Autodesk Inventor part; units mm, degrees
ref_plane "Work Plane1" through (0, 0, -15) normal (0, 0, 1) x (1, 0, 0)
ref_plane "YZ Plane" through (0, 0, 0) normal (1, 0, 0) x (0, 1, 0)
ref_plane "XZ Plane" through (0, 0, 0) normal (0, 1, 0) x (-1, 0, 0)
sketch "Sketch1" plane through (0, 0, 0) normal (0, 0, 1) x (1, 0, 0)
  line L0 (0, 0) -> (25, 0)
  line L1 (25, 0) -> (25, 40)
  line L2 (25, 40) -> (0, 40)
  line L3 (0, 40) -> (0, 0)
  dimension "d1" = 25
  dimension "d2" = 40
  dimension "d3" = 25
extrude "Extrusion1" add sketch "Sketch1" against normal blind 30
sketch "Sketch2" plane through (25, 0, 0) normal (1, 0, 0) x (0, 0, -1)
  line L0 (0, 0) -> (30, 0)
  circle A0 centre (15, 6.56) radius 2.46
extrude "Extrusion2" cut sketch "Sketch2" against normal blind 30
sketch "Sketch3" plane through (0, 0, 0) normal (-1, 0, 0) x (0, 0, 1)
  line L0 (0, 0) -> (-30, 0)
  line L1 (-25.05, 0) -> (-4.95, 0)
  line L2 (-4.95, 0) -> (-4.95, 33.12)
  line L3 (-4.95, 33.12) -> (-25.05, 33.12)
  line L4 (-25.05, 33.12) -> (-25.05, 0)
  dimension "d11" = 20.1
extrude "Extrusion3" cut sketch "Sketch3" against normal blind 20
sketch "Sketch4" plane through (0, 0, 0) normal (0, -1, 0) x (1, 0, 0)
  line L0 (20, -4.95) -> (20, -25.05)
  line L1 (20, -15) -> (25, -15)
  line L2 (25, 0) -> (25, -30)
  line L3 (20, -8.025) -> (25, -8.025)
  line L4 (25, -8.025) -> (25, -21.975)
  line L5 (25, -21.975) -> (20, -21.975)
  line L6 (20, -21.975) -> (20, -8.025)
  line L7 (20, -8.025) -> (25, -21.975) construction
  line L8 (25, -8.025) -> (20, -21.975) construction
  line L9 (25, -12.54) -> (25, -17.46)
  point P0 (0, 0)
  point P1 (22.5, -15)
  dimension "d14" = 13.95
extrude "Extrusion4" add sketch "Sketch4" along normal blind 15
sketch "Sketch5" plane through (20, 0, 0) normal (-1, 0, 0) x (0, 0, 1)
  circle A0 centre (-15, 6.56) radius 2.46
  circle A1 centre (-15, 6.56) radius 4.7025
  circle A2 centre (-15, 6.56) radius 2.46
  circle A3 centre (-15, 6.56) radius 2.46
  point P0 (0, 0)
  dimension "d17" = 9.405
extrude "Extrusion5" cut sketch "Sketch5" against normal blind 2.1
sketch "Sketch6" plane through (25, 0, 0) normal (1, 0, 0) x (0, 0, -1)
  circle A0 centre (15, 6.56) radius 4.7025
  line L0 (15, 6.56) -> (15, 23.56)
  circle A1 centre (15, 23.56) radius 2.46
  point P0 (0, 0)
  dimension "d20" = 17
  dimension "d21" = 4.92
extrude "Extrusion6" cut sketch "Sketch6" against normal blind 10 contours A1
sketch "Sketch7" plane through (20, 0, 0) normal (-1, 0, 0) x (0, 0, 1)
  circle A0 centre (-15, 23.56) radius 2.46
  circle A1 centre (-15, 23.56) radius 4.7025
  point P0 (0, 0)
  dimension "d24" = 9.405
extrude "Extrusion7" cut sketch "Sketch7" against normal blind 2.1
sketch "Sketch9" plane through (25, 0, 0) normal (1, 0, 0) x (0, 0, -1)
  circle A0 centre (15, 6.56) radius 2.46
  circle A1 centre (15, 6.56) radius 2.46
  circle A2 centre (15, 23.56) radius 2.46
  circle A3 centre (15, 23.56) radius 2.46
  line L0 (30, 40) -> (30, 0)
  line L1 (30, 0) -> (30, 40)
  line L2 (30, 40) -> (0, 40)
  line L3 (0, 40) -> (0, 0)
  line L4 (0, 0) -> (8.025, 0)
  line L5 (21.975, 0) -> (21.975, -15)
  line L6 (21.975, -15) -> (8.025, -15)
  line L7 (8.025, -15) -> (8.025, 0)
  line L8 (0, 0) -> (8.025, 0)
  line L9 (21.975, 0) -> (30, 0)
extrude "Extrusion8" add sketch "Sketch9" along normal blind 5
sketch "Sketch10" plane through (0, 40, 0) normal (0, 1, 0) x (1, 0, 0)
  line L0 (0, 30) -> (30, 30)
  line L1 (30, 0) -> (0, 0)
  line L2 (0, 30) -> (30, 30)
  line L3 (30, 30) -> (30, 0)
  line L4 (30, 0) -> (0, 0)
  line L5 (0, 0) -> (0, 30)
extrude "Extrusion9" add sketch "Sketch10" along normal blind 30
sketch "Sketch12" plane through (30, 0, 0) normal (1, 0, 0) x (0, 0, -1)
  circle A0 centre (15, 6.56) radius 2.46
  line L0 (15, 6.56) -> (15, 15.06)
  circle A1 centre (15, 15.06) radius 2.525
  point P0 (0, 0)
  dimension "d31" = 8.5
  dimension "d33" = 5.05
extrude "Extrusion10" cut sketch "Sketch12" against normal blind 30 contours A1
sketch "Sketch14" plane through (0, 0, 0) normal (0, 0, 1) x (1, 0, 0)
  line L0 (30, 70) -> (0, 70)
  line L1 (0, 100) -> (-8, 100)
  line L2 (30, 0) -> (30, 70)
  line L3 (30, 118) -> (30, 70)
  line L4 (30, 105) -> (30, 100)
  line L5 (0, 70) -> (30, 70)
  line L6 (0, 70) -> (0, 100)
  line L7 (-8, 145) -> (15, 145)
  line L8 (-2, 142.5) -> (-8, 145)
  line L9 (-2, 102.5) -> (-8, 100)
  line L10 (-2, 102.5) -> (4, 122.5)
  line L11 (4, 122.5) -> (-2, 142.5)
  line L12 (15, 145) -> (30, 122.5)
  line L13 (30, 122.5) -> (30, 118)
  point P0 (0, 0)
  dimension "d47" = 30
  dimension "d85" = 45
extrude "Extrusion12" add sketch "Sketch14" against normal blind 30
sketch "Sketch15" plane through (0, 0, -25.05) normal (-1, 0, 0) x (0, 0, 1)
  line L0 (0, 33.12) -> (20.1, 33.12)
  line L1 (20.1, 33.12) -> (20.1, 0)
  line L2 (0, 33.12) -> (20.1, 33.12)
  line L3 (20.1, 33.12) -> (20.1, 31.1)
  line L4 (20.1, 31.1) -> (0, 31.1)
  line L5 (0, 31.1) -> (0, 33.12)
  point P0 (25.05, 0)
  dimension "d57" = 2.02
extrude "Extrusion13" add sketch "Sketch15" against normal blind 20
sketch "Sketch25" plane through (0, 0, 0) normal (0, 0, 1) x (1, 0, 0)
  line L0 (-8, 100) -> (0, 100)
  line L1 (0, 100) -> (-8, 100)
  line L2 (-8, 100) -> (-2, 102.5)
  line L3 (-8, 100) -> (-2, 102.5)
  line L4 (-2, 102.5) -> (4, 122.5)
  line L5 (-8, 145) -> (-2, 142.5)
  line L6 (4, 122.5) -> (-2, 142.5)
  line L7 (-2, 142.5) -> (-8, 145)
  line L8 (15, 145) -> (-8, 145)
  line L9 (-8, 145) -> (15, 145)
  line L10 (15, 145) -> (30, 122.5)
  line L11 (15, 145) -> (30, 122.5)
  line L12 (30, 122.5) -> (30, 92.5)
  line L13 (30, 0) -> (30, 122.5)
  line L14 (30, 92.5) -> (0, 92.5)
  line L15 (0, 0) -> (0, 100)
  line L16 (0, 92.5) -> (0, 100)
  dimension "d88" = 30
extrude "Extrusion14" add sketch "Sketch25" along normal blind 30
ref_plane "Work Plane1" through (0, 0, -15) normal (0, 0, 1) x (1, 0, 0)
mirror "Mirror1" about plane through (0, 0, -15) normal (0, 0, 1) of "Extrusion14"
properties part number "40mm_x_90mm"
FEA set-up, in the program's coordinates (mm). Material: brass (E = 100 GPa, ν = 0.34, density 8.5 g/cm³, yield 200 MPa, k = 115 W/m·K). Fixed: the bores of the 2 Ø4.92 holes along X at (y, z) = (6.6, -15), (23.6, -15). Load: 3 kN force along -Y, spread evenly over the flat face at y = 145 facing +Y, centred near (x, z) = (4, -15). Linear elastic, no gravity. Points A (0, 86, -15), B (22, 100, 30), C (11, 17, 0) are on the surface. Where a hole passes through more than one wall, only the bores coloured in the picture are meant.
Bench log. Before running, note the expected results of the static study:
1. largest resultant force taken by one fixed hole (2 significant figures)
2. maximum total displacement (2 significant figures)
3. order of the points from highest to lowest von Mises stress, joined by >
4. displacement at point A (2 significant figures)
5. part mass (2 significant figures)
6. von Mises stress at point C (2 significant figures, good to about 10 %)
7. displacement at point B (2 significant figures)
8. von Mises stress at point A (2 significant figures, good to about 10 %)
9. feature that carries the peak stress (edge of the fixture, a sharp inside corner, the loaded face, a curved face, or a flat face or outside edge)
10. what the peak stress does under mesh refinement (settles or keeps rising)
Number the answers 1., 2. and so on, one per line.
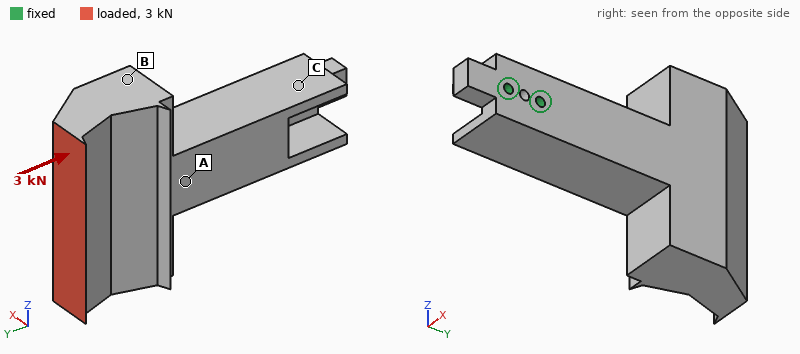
1. 3.1 kN
2. 0.16 mm
3. C > A > B
4. 0.077 mm
5. 1.7 kg
6. 19 MPa
7. 0.087 mm
8. 9.5 MPa
9. edge of the fixture
10. keeps rising
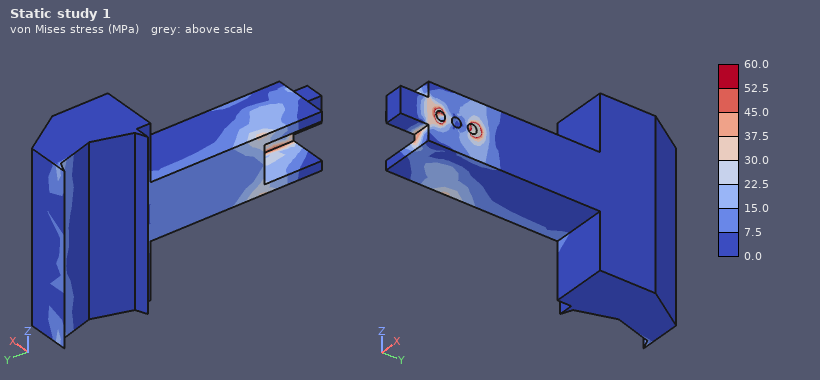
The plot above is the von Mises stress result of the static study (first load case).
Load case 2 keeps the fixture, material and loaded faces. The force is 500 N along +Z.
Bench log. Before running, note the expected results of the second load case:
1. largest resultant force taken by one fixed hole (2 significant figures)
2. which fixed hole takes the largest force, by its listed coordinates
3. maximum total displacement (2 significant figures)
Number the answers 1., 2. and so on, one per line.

1. 3.1 kN
2. (23.6, -15)
3. 0.13 mm
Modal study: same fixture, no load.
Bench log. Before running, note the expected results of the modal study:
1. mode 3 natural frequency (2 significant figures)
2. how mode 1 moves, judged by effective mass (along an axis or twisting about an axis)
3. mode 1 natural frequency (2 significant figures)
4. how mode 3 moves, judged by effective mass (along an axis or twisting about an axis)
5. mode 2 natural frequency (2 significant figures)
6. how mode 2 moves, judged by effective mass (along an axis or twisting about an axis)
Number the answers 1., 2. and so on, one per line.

1. 780 Hz
2. along X
3. 350 Hz
4. twisting about Y
5. 400 Hz
6. along Z
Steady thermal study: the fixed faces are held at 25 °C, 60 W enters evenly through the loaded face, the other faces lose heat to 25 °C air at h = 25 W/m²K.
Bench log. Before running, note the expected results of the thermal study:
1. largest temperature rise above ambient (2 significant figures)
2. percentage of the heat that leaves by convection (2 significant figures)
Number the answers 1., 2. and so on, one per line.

1. 56 K
2. 38 %
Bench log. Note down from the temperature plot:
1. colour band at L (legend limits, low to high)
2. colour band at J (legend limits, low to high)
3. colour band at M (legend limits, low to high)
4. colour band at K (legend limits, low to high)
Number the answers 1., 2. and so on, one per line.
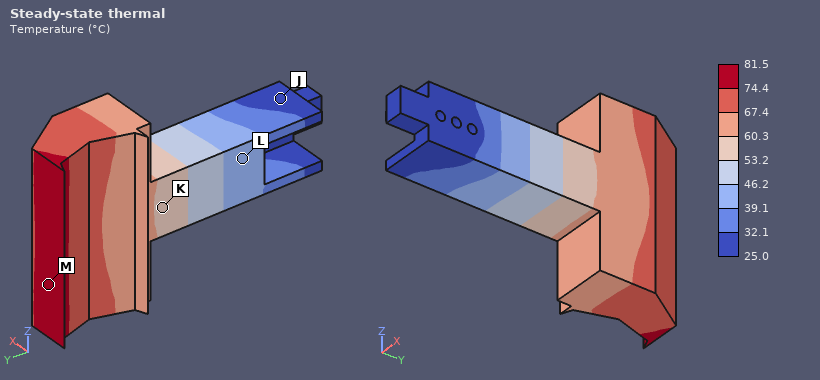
1. 39.1 to 46.2 °C
2. 25.0 to 32.1 °C
3. 74.4 to 81.5 °C
4. 53.2 to 60.3 °C
